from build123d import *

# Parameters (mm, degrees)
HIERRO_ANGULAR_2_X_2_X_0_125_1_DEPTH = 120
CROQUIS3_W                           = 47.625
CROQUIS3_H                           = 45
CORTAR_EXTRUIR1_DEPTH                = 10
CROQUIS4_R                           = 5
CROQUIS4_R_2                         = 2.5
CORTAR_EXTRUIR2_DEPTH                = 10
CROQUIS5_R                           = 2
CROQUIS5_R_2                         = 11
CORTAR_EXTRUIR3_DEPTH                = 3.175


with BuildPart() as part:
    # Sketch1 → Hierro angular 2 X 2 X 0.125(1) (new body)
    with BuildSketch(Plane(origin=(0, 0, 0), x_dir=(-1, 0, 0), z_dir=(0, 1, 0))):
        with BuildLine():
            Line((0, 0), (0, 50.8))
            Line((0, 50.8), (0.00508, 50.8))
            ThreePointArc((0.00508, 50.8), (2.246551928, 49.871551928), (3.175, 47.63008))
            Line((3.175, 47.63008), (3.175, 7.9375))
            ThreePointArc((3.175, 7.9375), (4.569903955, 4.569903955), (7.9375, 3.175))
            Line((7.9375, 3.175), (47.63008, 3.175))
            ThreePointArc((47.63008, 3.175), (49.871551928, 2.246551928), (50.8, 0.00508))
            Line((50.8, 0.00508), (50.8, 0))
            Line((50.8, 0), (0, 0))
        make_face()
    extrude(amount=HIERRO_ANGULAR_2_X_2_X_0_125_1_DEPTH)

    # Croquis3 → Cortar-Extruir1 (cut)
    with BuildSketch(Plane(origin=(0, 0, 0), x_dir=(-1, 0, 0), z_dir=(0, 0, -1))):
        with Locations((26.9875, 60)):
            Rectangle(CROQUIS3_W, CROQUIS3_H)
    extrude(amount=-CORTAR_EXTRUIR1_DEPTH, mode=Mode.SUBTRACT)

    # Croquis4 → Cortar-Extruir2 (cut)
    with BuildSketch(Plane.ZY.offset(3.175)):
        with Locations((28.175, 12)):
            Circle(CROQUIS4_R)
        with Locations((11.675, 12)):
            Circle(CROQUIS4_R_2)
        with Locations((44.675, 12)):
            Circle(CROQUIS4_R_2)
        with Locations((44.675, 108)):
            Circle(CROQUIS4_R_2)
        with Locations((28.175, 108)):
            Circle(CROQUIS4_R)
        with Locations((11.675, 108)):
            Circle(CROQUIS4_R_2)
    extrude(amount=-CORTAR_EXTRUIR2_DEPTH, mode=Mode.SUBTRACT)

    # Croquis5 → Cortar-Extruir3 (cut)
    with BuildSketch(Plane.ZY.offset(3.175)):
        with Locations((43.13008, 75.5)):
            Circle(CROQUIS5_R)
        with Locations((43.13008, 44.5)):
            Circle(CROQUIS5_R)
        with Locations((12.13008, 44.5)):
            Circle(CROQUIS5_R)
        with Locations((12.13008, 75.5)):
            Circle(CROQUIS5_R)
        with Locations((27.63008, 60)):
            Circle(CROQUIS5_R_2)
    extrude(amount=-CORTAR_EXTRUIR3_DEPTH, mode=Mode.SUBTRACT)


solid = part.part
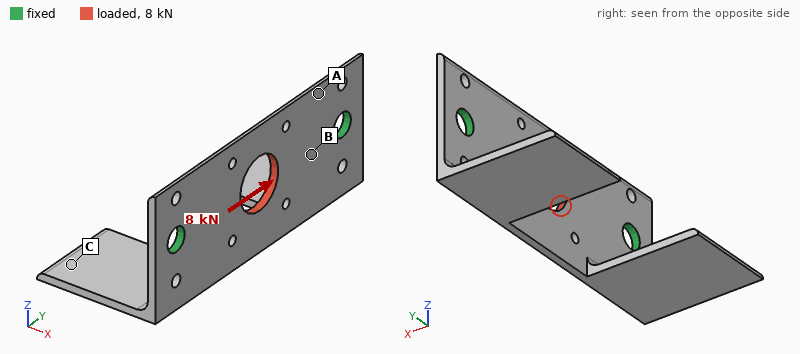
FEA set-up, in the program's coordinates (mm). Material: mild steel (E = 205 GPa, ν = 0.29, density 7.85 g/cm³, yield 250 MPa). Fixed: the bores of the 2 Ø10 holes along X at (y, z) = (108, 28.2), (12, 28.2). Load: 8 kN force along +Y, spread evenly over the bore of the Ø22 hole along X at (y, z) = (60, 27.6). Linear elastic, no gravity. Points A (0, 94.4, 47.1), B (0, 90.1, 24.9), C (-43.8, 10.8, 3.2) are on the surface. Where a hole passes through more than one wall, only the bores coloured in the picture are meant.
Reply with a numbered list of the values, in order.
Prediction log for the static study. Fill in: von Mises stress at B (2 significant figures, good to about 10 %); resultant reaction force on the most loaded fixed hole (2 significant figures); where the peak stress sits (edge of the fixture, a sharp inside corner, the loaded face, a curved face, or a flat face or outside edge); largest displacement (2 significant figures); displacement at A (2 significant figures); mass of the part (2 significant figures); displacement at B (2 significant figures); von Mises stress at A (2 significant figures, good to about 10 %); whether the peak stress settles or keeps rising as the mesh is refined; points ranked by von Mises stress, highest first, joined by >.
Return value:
1. 47 MPa
2. 4.0 kN
3. edge of the fixture
4. 8.9 µm
5. 4.0 µm
6. 220 g
7. 3.7 µm
8. 15 MPa
9. keeps rising
10. B > A > C
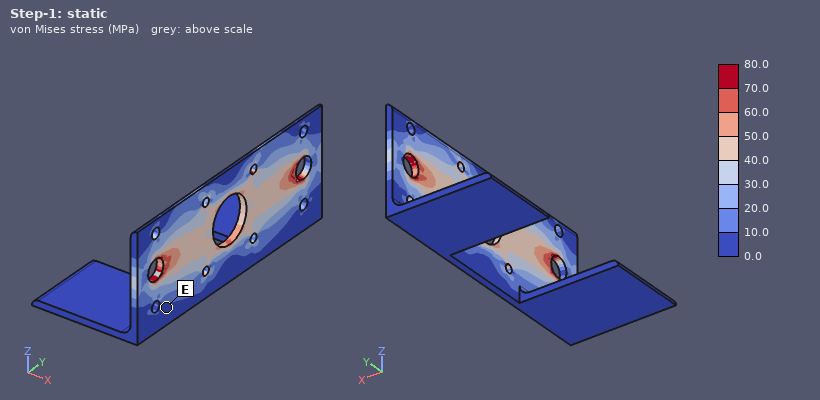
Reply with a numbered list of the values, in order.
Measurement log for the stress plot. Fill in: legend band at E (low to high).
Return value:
1. 0.0 to 10.0 MPa
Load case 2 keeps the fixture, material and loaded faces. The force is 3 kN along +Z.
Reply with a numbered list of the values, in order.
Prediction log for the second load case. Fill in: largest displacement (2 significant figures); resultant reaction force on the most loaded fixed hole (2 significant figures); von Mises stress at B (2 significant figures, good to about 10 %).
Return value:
1. 12 µm
2. 1.5 kN
3. 24 MPa
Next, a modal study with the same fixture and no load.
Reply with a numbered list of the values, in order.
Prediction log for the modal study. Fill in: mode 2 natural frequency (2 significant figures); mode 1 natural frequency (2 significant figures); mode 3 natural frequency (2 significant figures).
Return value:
1. 750 Hz
2. 670 Hz
3. 1100 Hz
